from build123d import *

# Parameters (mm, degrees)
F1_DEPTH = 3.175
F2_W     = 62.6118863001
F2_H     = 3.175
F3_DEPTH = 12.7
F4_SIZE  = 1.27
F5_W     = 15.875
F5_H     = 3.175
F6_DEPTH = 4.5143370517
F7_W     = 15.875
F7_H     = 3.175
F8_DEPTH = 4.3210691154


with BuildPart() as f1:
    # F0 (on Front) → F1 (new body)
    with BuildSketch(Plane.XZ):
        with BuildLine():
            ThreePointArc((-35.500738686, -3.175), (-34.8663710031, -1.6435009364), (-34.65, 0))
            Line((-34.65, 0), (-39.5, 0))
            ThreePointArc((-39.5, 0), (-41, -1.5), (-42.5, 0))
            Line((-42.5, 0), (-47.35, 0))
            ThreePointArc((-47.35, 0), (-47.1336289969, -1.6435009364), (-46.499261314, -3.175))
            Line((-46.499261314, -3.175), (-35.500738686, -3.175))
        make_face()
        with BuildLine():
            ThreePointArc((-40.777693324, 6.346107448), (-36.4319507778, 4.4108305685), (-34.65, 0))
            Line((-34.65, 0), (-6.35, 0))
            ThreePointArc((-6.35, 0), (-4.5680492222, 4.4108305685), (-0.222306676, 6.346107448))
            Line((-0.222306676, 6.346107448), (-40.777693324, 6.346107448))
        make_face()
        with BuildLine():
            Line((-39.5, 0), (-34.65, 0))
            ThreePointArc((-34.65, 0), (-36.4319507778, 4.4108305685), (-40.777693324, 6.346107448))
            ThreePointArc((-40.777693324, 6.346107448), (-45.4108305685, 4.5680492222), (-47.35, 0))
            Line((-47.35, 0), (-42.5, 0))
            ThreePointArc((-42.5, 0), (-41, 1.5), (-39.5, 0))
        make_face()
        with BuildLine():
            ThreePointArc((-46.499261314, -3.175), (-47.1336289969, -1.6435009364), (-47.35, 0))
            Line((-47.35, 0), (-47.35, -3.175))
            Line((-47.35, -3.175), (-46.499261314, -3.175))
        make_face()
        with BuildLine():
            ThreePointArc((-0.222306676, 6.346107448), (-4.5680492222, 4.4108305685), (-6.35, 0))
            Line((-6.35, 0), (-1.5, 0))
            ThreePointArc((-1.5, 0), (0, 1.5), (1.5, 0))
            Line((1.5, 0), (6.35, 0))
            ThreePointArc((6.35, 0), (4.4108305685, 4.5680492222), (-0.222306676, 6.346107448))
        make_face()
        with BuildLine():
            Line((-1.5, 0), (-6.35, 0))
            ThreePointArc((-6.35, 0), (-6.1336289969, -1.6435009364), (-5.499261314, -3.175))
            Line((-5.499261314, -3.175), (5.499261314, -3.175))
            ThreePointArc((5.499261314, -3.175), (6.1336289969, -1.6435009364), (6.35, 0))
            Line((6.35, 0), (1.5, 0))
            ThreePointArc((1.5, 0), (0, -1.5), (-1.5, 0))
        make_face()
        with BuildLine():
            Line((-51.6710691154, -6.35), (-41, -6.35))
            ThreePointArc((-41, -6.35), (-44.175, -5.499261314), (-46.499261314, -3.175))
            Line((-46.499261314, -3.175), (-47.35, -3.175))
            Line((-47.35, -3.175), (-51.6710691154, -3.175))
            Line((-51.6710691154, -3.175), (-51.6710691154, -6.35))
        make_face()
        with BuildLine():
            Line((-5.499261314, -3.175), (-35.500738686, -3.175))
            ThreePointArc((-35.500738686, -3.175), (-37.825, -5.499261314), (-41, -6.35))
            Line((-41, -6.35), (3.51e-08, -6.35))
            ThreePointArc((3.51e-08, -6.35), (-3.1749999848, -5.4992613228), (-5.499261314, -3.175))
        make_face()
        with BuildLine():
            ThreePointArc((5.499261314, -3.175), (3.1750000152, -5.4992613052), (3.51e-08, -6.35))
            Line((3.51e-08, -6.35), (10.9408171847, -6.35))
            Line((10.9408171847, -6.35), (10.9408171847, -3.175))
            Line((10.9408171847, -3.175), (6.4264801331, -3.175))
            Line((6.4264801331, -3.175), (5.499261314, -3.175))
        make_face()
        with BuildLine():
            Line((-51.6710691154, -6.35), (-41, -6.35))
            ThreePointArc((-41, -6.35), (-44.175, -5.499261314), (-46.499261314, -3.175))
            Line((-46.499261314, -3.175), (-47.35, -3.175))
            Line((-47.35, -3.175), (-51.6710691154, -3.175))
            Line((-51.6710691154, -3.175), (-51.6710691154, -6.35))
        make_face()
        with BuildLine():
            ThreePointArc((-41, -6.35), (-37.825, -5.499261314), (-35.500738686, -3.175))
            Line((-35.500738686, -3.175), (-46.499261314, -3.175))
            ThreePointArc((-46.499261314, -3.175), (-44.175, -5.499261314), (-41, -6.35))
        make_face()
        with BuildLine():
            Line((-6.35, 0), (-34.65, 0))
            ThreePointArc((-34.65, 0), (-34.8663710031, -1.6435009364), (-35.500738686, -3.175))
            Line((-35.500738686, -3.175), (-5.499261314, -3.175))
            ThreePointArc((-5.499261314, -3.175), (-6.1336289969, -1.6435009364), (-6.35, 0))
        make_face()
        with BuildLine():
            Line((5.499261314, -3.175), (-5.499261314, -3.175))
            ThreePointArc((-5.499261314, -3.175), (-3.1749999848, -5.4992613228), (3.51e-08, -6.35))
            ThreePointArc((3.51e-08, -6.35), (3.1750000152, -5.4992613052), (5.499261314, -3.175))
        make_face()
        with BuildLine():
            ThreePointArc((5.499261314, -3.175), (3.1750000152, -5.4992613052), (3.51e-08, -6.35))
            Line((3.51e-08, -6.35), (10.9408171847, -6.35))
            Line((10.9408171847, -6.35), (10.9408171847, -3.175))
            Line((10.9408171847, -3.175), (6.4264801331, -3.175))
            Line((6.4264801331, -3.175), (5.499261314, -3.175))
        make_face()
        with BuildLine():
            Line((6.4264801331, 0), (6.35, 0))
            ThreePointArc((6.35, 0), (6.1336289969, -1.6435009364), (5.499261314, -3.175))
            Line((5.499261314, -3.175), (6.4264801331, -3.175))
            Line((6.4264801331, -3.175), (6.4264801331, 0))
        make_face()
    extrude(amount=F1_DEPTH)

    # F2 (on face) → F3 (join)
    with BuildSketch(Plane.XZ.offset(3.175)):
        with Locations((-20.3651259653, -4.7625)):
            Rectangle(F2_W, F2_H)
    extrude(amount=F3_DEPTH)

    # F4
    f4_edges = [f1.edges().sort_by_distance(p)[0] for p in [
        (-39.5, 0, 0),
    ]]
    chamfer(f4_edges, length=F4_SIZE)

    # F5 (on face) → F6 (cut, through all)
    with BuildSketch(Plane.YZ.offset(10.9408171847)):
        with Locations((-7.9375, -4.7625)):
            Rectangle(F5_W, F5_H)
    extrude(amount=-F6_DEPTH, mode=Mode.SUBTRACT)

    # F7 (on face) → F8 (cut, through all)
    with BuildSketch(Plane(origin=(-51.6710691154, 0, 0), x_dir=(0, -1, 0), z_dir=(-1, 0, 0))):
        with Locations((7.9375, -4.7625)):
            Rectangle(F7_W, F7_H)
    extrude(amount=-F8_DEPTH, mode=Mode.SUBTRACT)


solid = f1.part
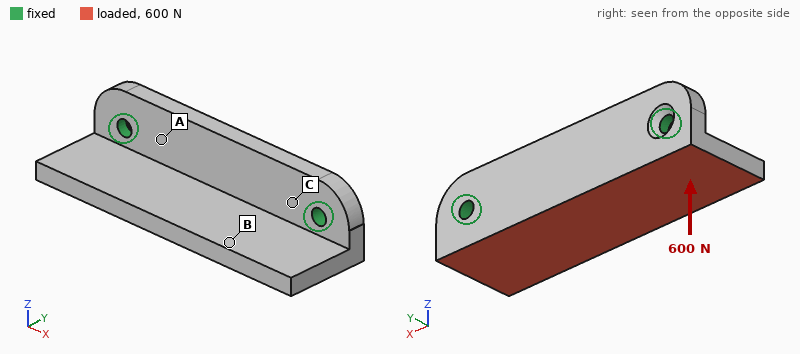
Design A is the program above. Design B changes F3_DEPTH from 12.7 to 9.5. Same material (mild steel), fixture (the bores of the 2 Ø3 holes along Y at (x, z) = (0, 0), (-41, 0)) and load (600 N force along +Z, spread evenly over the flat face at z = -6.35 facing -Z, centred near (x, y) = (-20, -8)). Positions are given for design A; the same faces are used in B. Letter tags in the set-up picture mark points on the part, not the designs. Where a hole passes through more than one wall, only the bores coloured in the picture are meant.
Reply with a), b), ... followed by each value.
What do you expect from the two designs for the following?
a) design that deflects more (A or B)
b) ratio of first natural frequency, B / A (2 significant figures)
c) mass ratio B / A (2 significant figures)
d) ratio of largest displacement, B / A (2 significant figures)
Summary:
a) A
b) 1.4
c) 0.87
d) 0.62
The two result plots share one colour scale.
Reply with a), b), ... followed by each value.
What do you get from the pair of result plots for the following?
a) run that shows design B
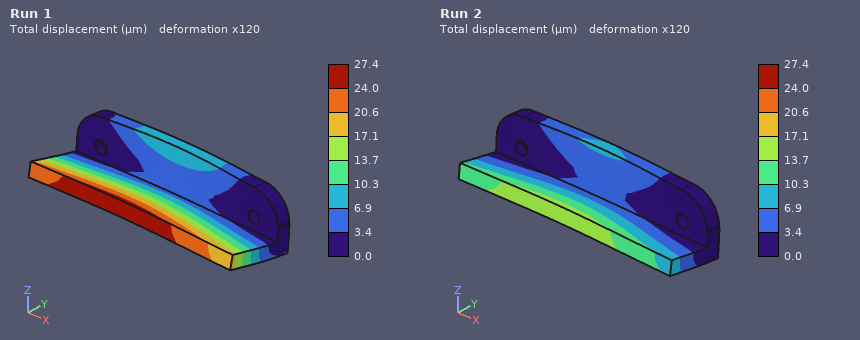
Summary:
a) Run 2
